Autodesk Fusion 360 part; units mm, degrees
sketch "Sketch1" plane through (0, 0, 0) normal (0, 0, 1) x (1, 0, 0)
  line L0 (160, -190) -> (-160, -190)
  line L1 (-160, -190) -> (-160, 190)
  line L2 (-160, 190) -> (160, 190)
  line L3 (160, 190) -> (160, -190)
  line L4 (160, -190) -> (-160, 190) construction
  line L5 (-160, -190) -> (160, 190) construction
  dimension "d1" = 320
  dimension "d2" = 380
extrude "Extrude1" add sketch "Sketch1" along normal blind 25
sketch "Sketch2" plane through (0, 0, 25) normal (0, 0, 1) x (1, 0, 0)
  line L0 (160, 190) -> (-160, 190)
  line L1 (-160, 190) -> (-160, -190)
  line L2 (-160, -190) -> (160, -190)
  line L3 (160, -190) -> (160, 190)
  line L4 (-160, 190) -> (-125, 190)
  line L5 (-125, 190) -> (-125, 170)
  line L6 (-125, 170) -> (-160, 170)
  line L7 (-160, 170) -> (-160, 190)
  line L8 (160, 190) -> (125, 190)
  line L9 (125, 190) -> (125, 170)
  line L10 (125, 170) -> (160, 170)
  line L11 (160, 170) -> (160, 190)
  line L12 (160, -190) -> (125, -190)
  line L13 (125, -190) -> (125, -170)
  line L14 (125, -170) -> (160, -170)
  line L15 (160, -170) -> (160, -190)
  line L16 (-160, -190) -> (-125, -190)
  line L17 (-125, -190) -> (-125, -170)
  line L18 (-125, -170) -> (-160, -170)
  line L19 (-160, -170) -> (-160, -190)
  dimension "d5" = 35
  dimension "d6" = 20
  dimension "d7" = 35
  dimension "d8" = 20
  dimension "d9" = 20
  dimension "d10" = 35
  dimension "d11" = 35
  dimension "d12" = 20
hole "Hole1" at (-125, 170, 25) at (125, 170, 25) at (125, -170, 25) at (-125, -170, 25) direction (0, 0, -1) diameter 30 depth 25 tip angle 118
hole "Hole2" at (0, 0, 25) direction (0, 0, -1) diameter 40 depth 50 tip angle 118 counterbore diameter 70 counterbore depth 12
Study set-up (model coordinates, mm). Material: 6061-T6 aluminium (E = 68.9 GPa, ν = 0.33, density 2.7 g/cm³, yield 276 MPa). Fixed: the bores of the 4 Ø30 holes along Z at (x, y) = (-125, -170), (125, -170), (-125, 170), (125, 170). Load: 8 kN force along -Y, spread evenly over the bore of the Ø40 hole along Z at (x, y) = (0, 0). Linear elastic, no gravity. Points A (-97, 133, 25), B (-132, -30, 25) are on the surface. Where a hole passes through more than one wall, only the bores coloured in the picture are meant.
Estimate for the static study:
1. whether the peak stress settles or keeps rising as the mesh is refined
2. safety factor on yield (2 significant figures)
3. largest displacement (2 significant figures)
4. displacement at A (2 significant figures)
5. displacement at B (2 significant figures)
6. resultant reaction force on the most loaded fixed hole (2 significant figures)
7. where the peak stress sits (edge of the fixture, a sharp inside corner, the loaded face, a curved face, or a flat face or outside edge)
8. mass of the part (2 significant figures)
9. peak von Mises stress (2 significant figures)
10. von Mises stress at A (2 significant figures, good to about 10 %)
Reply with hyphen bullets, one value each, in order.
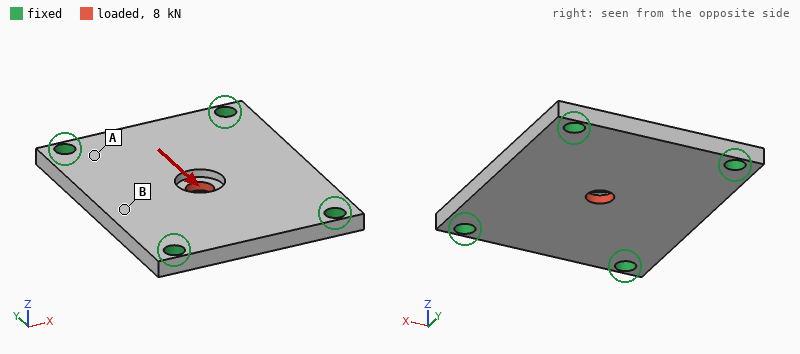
- settles
- 31
- 5.2 µm
- 0.96 µm
- 0.97 µm
- 2.2 kN
- the loaded face
- 7.8 kg
- 8.8 MPa
- 1.3 MPa
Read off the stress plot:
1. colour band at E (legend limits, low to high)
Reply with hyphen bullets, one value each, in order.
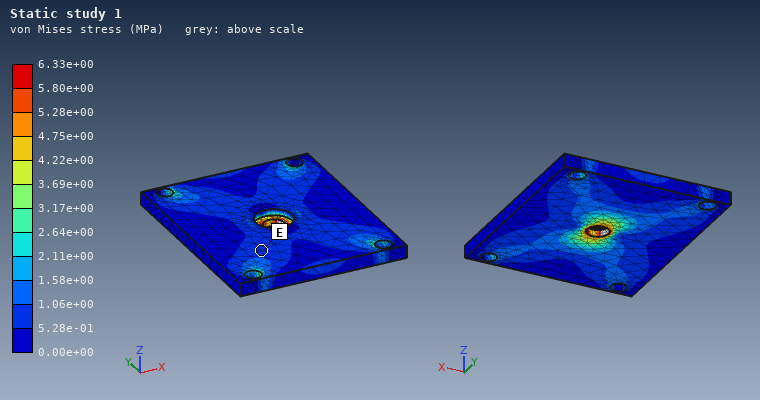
- 5.28e-01 to 1.06e+00 MPa
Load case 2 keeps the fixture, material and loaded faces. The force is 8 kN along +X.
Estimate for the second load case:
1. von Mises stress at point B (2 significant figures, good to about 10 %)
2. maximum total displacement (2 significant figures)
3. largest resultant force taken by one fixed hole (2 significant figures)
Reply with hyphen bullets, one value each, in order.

- 0.79 MPa
- 6.6 µm
- 2.4 kN
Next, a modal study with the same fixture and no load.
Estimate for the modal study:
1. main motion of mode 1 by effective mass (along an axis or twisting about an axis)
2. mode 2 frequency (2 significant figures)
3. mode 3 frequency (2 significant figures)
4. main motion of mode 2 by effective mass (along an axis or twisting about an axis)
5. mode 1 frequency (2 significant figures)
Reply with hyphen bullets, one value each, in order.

- along Z
- 1400 Hz
- 1900 Hz
- twisting about Y
- 950 Hz
